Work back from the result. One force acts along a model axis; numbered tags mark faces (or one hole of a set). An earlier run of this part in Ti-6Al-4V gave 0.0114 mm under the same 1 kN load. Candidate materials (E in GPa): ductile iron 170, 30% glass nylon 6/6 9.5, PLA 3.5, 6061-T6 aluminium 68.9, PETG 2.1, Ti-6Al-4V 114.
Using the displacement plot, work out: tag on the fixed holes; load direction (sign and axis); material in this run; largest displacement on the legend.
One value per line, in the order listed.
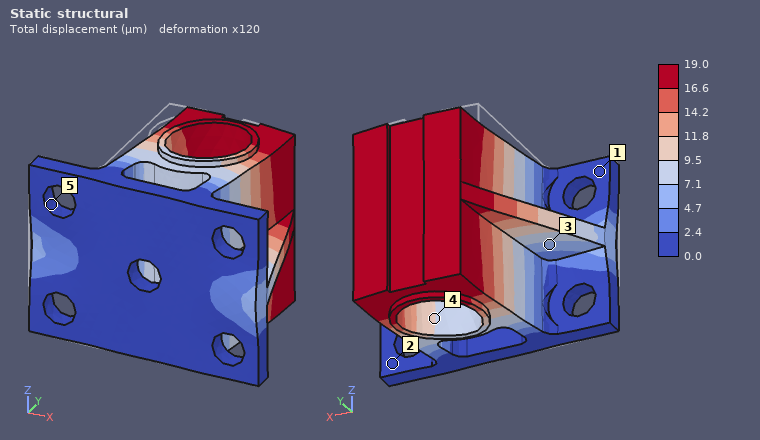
5
+X
6061-T6 aluminium
19.0 µm
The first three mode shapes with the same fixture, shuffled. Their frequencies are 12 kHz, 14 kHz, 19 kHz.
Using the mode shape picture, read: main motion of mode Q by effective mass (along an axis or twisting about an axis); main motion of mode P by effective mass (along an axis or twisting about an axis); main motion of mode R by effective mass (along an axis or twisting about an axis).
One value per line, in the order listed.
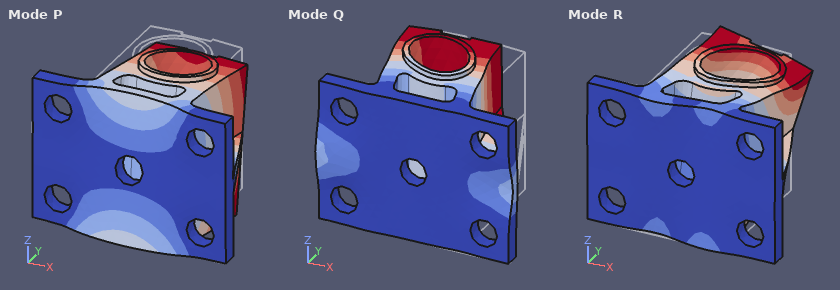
along X
along Z
twisting about Y
